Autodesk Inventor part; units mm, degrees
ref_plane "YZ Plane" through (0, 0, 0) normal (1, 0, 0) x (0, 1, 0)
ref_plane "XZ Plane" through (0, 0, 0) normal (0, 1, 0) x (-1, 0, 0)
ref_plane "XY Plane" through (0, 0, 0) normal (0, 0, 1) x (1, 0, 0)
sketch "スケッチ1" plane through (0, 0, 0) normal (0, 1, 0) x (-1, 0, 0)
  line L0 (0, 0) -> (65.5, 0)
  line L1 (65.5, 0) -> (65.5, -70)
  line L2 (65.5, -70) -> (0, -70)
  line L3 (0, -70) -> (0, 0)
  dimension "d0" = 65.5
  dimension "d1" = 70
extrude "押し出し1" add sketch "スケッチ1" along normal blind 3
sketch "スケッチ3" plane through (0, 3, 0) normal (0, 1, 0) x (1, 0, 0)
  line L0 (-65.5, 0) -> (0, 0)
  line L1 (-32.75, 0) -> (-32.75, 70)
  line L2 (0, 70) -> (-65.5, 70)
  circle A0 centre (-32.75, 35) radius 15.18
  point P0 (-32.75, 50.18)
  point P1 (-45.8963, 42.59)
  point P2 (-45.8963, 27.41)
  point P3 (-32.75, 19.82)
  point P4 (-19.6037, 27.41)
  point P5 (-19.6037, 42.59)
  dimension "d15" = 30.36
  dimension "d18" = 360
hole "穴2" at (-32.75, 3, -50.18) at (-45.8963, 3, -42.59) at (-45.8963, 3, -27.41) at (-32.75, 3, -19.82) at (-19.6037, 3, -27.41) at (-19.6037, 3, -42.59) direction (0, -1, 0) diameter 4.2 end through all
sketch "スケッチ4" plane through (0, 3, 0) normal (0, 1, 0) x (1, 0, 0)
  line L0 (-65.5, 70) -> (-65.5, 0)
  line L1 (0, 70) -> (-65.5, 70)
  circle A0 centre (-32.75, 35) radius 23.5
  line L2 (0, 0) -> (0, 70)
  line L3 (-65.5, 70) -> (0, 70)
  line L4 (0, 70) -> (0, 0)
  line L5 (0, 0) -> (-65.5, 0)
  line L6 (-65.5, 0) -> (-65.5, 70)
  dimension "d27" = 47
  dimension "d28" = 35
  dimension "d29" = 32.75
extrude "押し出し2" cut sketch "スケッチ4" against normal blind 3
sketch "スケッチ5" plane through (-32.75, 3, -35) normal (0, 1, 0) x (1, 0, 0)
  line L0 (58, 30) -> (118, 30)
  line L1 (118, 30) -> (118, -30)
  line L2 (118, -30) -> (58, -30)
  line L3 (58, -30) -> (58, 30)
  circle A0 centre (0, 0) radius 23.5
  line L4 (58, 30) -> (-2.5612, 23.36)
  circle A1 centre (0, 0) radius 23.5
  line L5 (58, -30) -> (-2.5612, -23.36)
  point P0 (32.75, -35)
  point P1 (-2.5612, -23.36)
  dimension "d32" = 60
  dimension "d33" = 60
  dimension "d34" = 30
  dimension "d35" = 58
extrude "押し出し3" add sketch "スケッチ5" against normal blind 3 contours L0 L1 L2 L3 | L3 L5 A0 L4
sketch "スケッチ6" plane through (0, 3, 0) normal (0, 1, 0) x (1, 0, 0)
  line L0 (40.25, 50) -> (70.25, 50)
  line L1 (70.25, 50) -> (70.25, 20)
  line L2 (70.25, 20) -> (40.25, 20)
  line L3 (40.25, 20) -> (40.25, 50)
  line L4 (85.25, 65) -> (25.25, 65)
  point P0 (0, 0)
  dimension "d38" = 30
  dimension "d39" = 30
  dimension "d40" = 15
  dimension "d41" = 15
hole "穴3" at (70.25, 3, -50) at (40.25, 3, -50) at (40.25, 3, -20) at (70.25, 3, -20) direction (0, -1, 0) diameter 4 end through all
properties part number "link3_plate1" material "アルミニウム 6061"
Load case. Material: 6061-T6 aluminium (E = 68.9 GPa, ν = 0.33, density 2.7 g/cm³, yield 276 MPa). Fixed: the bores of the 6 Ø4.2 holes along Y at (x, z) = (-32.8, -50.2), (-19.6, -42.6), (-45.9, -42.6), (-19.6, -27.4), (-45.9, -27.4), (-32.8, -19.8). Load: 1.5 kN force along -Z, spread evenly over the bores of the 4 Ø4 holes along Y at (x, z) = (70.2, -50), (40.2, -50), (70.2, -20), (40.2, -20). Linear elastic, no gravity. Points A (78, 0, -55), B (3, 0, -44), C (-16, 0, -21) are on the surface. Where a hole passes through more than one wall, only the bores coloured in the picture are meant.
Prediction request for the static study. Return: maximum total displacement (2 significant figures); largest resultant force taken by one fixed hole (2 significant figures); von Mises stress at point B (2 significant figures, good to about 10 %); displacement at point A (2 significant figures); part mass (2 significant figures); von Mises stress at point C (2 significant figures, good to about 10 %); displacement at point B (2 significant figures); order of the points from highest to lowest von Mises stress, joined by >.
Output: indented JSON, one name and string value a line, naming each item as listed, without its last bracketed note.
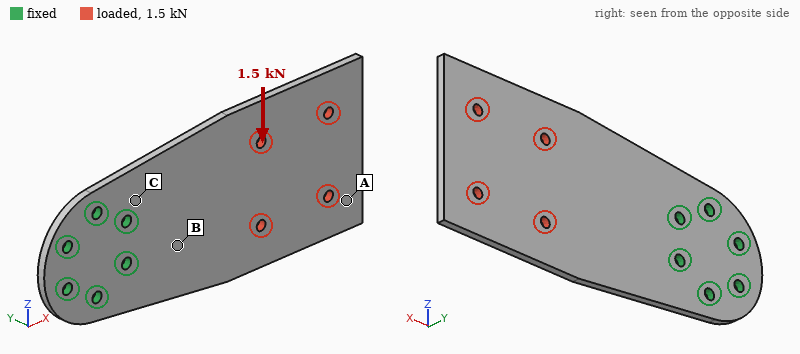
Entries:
{
  "maximum total displacement": "0.24 mm",
  "largest resultant force taken by one fixed hole": "2.3 kN",
  "von Mises stress at point B": "32 MPa",
  "displacement at point A": "0.22 mm",
  "part mass": "60 g",
  "von Mises stress at point C": "48 MPa",
  "displacement at point B": "0.039 mm",
  "order of the points from highest to lowest von Mises stress, joined by >": "C > B > A"
}
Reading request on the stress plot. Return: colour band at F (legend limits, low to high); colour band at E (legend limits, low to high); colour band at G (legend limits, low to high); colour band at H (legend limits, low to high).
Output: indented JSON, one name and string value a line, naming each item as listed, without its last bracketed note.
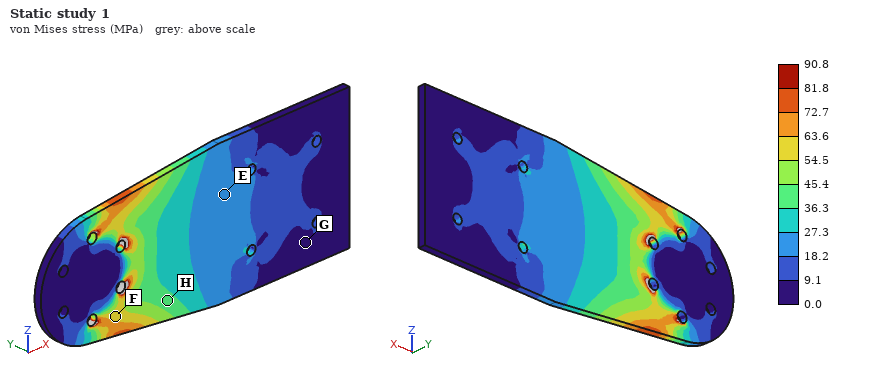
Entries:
{
  "colour band at F": "54.5 to 63.6 MPa",
  "colour band at E": "18.2 to 27.3 MPa",
  "colour band at G": "0.0 to 9.1 MPa",
  "colour band at H": "36.3 to 45.4 MPa"
}
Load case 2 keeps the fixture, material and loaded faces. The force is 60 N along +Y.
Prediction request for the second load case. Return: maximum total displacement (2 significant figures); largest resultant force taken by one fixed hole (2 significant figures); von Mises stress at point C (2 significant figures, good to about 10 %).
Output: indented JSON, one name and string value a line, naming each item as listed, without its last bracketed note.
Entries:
{
  "maximum total displacement": "1.5 mm",
  "largest resultant force taken by one fixed hole": "98 N",
  "von Mises stress at point C": "46 MPa"
}
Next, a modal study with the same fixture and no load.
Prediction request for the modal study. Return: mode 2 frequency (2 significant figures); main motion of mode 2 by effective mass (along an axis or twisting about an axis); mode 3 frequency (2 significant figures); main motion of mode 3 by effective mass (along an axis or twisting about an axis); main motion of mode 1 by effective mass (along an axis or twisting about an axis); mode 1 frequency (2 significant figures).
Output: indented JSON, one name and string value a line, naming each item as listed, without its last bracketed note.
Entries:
{
  "mode 2 frequency": "770 Hz",
  "main motion of mode 2 by effective mass": "twisting about X",
  "mode 3 frequency": "1400 Hz",
  "main motion of mode 3 by effective mass": "along Y",
  "main motion of mode 1 by effective mass": "along Y",
  "mode 1 frequency": "220 Hz"
}
